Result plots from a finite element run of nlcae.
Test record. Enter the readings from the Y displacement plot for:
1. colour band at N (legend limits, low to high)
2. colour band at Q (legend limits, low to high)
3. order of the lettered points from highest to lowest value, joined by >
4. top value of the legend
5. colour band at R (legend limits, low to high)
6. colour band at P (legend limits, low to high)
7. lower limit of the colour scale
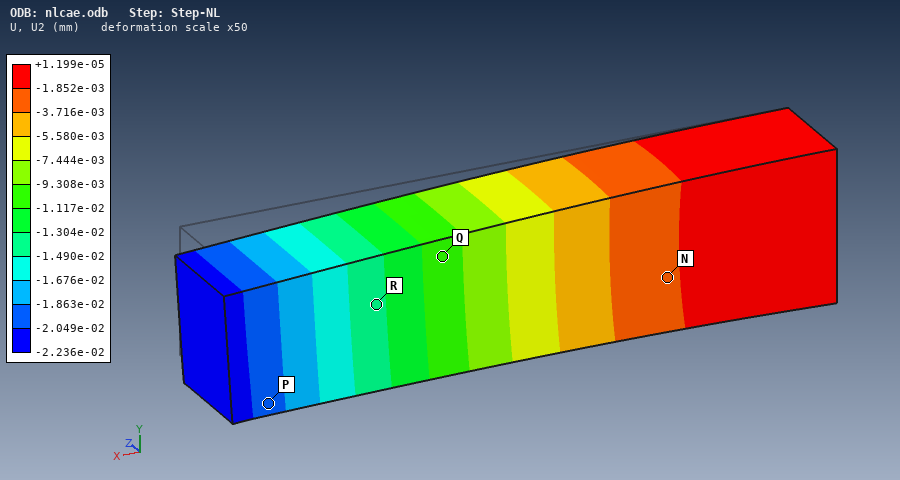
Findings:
-3.716e-03 to -1.852e-03 mm
-1.117e-02 to -9.308e-03 mm
N > Q > R > P
+1.199e-05 mm
-1.490e-02 to -1.304e-02 mm
-2.049e-02 to -1.863e-02 mm
-2.236e-02 mm
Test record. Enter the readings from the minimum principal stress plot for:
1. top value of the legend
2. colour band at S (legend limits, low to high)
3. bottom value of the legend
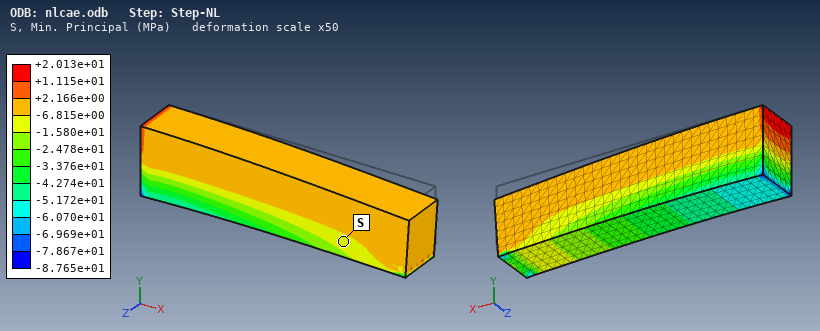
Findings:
+2.013e+01 MPa
-1.580e+01 to -6.815e+00 MPa
-8.765e+01 MPa
